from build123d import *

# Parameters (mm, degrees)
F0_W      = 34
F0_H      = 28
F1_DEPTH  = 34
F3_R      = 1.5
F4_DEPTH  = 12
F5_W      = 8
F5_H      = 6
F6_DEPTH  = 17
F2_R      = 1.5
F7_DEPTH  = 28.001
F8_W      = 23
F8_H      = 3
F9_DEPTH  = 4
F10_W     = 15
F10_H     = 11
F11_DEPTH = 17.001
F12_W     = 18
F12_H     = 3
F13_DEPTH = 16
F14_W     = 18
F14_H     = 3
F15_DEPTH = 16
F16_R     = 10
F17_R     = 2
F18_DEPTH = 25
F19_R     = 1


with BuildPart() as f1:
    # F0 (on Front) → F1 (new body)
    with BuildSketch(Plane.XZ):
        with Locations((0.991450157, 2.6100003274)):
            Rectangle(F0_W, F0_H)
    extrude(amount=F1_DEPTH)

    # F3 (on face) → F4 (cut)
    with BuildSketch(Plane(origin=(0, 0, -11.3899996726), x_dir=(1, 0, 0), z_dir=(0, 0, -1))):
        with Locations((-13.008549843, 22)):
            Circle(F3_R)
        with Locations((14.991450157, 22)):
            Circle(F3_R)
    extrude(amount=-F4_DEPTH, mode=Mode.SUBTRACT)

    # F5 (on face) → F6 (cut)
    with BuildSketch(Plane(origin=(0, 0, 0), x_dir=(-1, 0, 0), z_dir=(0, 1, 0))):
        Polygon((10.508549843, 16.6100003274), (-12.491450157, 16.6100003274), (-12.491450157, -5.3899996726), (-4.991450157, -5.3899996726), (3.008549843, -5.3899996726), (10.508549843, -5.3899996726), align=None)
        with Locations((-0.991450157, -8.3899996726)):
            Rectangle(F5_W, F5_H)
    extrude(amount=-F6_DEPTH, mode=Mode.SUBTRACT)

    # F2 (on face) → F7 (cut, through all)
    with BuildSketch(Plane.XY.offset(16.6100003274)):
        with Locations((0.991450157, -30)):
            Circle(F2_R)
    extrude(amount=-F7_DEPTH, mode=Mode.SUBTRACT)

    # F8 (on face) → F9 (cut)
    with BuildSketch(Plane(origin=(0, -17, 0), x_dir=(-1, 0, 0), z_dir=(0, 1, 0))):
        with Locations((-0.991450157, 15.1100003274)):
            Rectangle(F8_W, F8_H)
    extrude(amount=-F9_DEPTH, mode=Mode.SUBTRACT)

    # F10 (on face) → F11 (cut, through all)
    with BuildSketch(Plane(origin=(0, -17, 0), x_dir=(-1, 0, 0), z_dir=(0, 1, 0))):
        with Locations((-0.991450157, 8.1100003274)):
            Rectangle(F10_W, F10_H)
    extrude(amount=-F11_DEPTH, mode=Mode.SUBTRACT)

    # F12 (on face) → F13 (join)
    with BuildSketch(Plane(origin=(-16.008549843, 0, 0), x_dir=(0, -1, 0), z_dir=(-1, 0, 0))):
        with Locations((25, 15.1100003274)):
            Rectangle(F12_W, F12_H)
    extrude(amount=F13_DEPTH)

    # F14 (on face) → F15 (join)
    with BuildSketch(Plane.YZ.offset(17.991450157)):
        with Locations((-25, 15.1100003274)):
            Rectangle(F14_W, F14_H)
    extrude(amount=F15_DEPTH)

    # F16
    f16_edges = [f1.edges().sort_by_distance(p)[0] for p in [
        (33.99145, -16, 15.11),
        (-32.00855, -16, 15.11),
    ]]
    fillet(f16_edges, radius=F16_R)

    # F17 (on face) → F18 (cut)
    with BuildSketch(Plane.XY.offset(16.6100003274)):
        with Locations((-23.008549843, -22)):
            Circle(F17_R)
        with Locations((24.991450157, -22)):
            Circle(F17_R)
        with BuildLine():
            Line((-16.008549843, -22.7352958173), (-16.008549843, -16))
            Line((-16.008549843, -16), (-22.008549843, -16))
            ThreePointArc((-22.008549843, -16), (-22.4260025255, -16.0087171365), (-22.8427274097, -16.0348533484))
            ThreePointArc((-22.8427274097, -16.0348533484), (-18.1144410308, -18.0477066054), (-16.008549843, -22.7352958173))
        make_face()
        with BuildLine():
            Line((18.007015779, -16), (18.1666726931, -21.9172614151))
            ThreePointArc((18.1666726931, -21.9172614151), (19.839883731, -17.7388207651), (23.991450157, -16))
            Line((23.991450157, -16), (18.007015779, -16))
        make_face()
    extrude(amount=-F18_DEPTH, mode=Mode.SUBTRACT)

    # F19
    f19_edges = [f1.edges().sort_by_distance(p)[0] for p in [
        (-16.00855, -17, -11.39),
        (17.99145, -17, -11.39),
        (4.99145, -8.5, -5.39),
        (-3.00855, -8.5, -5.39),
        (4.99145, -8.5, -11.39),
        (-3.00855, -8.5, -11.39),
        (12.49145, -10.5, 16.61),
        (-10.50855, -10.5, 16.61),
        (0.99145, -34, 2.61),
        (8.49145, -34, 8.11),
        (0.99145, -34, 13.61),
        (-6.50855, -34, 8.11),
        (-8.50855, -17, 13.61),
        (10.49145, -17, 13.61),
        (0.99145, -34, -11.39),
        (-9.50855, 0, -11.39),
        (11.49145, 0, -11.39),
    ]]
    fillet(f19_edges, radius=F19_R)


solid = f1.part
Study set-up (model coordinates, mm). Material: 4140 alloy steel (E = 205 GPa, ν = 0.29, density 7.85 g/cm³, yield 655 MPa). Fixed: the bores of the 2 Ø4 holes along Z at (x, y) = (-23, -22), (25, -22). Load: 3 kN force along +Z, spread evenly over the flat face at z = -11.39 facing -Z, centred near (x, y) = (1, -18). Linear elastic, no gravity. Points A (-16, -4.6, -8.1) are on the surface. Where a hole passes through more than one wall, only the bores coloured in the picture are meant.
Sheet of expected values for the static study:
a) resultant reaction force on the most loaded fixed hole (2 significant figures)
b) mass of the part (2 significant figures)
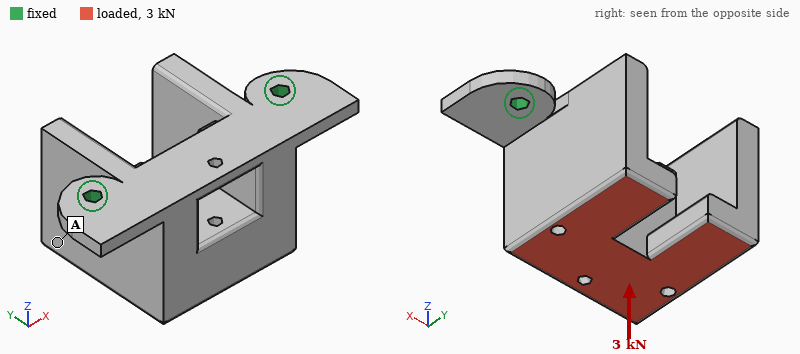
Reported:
1.6 kN
160 g
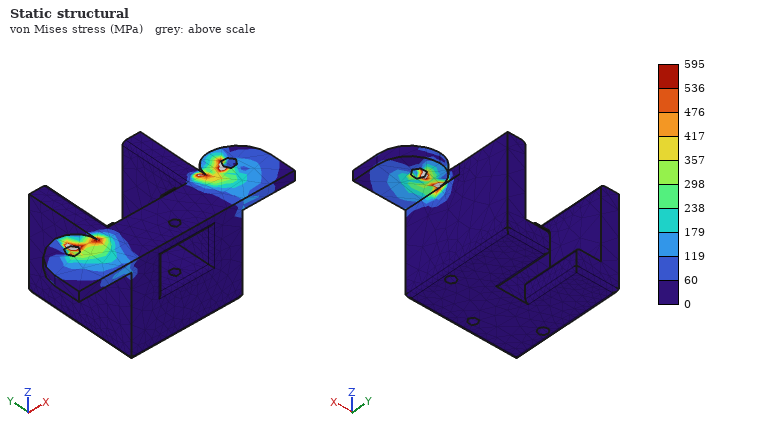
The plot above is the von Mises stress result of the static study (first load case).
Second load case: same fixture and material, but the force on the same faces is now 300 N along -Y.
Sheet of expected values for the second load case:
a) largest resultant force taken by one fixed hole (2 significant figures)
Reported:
190 N
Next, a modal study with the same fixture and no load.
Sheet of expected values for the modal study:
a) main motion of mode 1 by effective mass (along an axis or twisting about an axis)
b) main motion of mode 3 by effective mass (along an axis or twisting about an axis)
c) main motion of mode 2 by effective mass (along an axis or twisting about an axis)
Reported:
along Y
along Z
along X
